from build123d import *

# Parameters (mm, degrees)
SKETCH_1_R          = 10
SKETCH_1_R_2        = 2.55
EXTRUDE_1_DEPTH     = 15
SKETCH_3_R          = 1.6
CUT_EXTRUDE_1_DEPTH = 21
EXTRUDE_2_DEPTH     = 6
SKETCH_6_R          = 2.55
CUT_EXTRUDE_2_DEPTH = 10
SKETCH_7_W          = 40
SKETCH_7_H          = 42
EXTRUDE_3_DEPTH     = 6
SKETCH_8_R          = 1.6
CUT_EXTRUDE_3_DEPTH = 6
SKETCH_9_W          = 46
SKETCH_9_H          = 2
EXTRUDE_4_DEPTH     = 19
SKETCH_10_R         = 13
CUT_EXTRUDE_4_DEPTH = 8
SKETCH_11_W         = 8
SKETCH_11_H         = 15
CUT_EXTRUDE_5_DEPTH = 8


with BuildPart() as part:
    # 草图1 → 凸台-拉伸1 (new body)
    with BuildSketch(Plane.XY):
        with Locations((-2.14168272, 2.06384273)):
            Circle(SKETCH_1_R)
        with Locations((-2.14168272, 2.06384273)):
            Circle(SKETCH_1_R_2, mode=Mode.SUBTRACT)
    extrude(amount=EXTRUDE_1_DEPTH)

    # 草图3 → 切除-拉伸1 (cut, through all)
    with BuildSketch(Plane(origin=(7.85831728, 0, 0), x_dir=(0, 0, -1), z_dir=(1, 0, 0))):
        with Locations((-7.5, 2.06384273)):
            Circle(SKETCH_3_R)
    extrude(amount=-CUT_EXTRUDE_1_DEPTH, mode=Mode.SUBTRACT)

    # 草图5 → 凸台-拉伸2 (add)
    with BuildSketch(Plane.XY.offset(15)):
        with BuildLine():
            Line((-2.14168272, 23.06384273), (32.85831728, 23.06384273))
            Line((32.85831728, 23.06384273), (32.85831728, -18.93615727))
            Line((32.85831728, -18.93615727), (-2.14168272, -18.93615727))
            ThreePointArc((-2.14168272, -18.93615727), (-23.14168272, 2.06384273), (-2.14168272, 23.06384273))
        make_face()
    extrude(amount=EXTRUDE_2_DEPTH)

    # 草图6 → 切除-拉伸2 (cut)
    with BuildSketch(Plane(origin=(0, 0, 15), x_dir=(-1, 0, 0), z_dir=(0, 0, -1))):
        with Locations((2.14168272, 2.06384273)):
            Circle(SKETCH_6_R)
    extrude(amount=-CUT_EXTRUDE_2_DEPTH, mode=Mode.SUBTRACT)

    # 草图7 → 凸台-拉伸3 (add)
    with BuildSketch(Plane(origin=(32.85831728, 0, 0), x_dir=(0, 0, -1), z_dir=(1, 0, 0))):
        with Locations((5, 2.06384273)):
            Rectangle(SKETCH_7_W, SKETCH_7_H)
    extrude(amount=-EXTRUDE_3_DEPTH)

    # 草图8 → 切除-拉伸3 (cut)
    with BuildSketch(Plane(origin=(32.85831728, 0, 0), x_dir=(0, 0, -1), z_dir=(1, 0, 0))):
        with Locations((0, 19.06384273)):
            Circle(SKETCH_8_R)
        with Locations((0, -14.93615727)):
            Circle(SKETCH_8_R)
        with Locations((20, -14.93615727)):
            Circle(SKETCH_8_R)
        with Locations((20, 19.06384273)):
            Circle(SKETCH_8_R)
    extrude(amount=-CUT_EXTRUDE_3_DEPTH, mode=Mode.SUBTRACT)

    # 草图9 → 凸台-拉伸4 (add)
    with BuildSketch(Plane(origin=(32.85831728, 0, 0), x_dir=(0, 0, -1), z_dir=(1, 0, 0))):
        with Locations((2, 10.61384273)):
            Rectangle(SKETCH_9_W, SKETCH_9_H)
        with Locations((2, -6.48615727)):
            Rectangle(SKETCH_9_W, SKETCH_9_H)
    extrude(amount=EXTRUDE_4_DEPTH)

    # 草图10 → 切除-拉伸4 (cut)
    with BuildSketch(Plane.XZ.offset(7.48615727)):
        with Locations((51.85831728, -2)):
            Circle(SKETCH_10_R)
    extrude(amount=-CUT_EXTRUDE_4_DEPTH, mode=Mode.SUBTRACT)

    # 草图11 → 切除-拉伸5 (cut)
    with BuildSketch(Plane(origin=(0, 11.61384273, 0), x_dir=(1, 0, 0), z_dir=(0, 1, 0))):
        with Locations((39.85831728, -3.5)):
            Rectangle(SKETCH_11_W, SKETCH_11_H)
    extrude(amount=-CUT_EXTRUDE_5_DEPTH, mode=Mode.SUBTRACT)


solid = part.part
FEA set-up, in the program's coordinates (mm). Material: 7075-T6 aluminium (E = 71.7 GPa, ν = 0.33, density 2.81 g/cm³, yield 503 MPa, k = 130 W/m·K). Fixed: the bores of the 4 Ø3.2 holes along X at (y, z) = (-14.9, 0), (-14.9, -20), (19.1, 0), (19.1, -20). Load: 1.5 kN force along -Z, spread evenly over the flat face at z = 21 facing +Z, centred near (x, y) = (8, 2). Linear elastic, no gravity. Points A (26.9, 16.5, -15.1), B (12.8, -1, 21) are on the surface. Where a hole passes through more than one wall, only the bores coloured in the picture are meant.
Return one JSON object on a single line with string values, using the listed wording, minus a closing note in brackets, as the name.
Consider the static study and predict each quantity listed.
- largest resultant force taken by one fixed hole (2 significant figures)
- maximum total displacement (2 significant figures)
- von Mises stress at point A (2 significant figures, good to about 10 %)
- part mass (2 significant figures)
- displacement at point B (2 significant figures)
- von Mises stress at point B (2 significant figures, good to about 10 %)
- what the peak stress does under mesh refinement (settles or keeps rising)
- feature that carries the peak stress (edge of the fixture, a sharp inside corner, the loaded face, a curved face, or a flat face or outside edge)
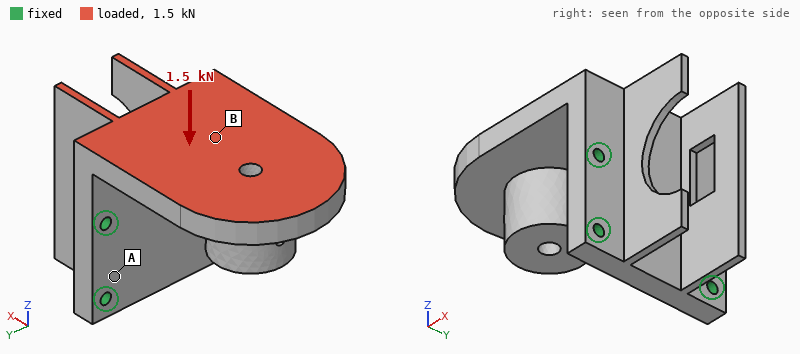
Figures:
{"largest resultant force taken by one fixed hole": "990 N", "maximum total displacement": "0.67 mm", "von Mises stress at point A": "16 MPa", "part mass": "84 g", "displacement at point B": "0.19 mm", "von Mises stress at point B": "50 MPa", "what the peak stress does under mesh refinement": "keeps rising", "feature that carries the peak stress": "edge of the fixture"}
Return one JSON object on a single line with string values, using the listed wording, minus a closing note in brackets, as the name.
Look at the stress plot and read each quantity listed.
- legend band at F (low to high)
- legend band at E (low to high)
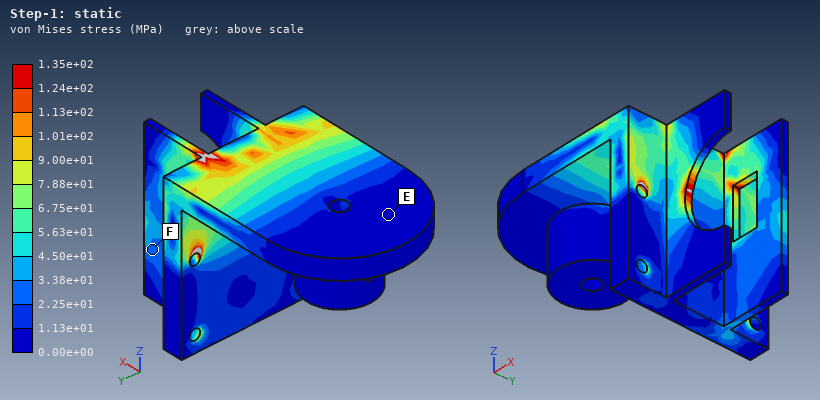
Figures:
{"legend band at F": "2.25e+01 to 3.38e+01 MPa", "legend band at E": "0.00e+00 to 1.13e+01 MPa"}
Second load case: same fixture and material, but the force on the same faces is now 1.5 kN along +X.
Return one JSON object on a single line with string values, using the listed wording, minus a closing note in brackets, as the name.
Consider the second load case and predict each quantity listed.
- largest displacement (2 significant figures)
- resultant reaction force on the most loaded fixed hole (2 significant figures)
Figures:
{"largest displacement": "0.27 mm", "resultant reaction force on the most loaded fixed hole": "1.2 kN"}
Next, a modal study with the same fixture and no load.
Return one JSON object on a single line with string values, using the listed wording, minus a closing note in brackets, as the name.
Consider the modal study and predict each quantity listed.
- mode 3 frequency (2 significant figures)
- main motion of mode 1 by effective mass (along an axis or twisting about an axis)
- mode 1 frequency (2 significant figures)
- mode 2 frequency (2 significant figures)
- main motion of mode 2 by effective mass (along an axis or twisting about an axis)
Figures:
{"mode 3 frequency": "3700 Hz", "main motion of mode 1 by effective mass": "along Z", "mode 1 frequency": "1300 Hz", "mode 2 frequency": "2400 Hz", "main motion of mode 2 by effective mass": "along Y"}
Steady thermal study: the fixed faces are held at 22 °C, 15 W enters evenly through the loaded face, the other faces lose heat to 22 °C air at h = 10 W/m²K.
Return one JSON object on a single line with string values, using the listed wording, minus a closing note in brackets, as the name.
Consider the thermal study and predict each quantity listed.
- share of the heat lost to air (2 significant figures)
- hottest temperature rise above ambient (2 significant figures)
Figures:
{"share of the heat lost to air": "5.4 %", "hottest temperature rise above ambient": "17 K"}
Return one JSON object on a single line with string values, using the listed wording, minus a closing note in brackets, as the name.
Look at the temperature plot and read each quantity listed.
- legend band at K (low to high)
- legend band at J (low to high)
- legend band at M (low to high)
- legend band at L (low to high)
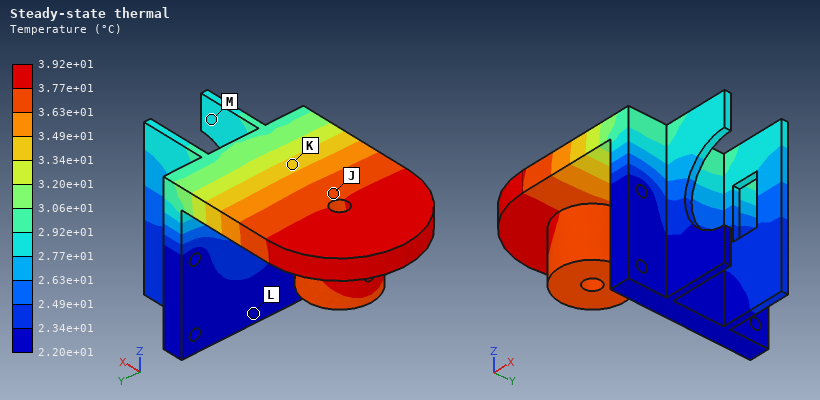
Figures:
{"legend band at K": "3.34e+01 to 3.49e+01 °C", "legend band at J": "3.63e+01 to 3.77e+01 °C", "legend band at M": "2.77e+01 to 2.92e+01 °C", "legend band at L": "2.20e+01 to 2.34e+01 °C"}
